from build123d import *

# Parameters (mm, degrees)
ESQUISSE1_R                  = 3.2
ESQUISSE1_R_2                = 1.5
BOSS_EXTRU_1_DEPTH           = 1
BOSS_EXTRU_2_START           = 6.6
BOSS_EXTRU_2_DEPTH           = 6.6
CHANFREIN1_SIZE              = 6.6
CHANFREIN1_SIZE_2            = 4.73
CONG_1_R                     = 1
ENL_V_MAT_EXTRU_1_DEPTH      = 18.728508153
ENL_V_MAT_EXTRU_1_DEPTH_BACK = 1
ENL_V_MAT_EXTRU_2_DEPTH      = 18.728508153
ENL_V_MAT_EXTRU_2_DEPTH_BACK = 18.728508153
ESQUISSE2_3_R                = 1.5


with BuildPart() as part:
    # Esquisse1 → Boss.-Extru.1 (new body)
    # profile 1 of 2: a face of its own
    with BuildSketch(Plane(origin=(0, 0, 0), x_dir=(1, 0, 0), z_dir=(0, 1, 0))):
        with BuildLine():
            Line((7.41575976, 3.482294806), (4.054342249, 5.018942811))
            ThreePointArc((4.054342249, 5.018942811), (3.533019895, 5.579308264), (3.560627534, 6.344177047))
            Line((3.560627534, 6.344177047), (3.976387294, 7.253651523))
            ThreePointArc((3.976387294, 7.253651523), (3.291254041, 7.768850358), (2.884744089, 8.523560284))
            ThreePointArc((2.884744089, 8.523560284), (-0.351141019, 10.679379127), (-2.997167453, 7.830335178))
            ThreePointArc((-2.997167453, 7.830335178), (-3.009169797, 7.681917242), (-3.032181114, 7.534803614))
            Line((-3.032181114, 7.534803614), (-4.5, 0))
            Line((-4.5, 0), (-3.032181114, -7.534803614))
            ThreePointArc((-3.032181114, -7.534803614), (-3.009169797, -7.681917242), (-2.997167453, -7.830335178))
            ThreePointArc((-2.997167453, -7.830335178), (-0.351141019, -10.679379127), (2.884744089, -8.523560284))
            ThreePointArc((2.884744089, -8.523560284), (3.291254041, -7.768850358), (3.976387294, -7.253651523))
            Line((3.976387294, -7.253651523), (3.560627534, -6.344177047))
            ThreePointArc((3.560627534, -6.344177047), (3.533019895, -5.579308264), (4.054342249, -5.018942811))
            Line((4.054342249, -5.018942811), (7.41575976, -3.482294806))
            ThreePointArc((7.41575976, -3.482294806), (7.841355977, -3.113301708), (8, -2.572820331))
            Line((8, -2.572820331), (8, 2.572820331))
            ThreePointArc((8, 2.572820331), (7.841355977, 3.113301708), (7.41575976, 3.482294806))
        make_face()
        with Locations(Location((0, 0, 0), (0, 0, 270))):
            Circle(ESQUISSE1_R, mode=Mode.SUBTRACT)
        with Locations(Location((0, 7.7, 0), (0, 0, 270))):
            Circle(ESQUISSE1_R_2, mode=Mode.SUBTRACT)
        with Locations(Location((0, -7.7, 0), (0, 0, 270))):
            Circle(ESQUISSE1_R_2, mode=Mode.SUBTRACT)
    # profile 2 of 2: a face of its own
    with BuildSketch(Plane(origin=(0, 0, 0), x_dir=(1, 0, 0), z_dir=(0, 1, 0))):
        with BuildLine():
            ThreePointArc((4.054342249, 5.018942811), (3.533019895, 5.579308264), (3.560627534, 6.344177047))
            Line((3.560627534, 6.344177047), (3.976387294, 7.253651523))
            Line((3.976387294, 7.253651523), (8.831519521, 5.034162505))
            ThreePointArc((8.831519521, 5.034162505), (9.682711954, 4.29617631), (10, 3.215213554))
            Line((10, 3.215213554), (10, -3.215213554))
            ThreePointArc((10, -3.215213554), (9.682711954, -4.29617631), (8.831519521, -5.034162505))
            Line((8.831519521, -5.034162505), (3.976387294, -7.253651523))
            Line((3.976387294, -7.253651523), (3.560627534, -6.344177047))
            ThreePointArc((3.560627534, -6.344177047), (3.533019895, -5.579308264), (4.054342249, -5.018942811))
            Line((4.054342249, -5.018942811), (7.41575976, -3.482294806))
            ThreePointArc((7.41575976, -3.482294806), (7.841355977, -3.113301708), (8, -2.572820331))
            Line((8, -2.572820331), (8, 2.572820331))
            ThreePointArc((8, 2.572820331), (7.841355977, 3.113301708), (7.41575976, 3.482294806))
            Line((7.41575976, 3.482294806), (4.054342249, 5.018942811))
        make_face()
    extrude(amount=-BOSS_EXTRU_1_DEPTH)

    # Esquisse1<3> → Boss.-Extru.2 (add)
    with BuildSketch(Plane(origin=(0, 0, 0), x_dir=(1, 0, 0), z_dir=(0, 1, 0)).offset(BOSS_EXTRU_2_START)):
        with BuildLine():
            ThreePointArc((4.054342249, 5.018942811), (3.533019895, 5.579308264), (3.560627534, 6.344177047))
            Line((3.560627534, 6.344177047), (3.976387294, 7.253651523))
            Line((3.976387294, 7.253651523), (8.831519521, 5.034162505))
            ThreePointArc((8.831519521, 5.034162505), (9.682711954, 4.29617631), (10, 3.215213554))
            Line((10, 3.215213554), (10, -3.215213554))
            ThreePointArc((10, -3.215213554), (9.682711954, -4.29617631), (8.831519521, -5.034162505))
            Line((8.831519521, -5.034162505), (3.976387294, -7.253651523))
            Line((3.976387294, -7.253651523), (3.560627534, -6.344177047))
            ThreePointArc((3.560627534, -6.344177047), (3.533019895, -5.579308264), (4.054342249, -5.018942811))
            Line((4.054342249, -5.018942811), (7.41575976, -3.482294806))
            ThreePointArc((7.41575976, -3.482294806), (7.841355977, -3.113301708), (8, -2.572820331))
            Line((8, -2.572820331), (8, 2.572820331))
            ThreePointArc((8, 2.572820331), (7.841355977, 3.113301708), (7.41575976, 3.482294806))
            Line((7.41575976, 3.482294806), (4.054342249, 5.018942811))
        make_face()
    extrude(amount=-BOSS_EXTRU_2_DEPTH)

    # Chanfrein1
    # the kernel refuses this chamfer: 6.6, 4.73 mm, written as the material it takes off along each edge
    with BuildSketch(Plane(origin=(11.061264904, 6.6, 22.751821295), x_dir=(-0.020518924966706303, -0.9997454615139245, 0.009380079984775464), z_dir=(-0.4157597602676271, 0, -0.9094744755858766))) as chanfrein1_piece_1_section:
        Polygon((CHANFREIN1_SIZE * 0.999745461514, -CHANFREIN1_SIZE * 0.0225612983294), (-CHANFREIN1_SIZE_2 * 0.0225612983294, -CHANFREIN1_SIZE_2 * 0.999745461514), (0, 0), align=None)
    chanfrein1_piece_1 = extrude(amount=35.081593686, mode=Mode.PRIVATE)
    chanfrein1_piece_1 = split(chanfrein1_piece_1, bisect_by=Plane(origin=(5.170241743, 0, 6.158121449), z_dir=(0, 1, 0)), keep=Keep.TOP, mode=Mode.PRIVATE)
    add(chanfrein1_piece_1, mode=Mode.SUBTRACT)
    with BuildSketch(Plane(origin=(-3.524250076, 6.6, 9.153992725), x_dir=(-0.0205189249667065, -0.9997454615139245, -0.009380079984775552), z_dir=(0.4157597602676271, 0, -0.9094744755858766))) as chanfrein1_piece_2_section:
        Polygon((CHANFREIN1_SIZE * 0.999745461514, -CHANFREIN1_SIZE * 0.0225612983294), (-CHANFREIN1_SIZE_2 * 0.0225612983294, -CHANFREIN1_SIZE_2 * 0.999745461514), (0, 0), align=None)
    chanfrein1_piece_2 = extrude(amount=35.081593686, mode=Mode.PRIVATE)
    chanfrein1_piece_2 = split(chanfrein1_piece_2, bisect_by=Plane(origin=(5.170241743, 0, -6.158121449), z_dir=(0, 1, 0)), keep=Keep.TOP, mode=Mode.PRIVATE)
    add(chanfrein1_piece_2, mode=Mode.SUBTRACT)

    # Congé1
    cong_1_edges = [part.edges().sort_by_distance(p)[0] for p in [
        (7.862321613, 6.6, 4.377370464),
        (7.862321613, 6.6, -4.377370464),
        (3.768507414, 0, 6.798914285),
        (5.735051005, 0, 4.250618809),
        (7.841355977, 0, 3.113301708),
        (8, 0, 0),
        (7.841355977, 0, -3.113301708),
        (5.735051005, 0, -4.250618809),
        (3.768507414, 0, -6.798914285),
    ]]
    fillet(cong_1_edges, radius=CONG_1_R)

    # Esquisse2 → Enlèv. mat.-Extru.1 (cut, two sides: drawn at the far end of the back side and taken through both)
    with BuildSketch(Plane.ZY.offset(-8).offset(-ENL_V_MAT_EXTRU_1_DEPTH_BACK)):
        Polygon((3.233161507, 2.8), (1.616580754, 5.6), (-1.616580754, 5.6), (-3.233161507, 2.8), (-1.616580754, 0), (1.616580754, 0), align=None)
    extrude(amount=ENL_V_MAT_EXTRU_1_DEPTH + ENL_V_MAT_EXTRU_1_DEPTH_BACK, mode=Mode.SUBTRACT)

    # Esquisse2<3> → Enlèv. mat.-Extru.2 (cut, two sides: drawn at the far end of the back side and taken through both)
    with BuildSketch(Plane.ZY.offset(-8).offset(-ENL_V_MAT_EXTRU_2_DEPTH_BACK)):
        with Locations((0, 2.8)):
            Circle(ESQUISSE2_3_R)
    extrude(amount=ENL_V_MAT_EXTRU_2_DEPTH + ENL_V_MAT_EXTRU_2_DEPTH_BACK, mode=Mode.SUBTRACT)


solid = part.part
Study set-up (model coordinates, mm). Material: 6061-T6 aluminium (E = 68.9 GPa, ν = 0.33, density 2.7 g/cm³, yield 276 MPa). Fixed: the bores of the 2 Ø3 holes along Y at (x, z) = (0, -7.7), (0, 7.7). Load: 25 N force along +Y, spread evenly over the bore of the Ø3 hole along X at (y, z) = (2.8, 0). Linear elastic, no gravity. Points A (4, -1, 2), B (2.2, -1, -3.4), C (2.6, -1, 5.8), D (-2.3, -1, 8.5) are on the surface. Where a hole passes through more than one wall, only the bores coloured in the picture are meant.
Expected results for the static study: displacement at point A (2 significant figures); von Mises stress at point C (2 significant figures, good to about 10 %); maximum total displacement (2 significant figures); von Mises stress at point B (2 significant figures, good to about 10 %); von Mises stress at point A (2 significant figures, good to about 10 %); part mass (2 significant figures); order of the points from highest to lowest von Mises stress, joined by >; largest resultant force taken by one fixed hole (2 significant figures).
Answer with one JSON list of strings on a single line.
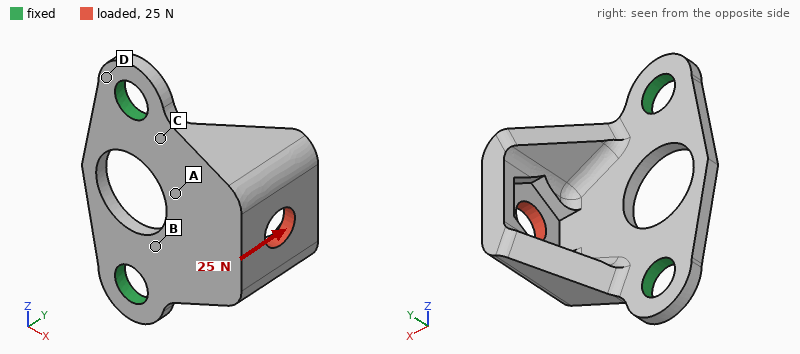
["18 µm", "85 MPa", "97 µm", "67 MPa", "24 MPa", "0.90 g", "C > B > A > D", "13 N"]
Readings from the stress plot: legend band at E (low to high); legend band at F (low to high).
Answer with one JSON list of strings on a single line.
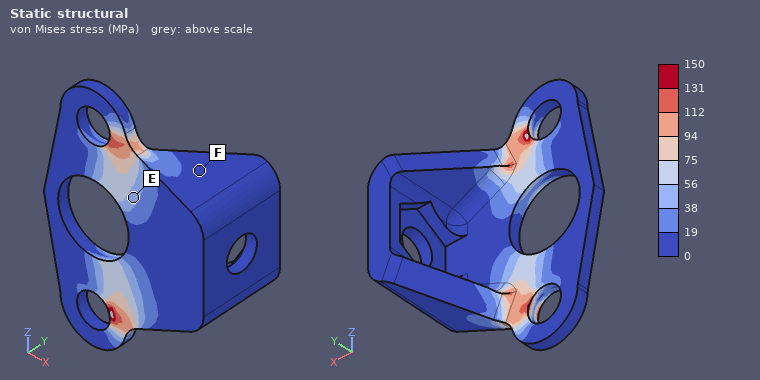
["38 to 56 MPa", "0 to 19 MPa"]
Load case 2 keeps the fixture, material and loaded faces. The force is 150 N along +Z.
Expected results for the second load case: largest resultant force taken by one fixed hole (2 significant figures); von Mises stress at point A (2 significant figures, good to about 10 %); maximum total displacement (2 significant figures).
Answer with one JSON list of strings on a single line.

["120 N", "16 MPa", "25 µm"]
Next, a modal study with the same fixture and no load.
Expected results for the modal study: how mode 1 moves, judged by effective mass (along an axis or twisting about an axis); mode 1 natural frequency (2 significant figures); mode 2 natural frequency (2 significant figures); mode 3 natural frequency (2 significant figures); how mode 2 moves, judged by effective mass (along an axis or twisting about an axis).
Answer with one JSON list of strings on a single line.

["along Y", "4400 Hz", "18 kHz", "31 kHz", "along Z"]
